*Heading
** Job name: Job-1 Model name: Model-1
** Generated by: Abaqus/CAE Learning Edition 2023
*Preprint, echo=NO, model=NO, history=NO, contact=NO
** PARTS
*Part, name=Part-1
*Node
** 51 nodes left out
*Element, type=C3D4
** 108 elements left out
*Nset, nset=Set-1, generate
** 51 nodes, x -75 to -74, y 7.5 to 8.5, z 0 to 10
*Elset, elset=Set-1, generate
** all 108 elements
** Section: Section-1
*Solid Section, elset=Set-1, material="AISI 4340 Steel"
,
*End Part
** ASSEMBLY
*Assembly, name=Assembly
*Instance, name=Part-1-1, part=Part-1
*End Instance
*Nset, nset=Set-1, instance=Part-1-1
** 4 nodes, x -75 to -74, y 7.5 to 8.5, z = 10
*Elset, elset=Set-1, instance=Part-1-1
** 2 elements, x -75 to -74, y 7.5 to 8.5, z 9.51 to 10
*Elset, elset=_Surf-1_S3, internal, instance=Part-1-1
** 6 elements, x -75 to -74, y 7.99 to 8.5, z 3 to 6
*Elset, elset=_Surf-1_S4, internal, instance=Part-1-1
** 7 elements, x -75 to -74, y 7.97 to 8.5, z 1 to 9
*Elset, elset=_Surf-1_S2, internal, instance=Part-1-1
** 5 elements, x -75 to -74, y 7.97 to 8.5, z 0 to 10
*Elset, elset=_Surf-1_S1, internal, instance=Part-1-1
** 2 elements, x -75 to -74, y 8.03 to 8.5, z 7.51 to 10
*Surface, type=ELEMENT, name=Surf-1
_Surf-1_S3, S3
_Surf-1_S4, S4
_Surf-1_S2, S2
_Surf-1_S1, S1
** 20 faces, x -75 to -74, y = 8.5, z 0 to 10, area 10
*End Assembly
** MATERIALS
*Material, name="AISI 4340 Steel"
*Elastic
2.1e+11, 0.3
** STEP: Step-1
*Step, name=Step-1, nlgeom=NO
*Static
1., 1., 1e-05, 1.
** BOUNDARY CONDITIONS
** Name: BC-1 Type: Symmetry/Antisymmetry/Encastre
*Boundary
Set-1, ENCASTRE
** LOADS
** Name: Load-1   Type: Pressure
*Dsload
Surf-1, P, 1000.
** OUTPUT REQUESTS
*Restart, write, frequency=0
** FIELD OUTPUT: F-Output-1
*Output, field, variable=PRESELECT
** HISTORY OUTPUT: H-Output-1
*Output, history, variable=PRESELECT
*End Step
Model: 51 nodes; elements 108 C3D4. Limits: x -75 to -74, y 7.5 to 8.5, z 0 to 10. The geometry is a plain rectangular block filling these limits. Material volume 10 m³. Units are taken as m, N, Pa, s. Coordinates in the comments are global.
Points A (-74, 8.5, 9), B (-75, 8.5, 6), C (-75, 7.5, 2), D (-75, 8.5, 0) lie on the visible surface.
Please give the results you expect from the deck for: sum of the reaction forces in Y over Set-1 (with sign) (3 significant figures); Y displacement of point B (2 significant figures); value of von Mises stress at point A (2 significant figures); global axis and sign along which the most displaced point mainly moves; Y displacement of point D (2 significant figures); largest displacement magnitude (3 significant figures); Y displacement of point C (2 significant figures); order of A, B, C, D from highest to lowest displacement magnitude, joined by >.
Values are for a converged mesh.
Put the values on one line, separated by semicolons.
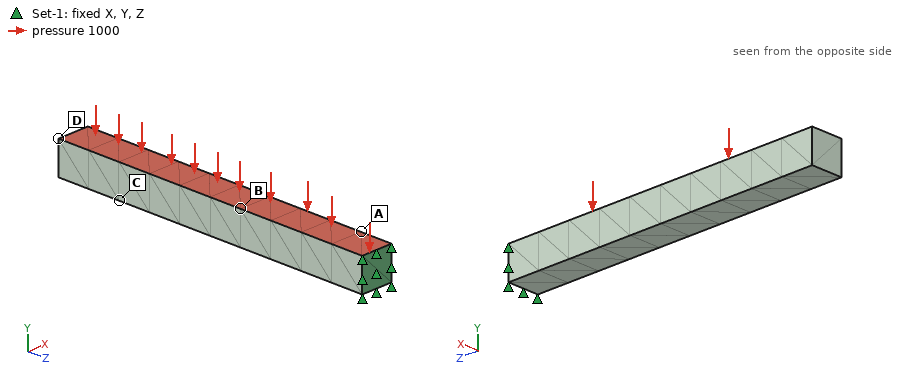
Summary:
10000 N; -1.7e-05 m; 2.4e+05 Pa; -Y; -7.1e-05 m; 7.15e-05 m; -5.2e-05 m; D > C > B > A
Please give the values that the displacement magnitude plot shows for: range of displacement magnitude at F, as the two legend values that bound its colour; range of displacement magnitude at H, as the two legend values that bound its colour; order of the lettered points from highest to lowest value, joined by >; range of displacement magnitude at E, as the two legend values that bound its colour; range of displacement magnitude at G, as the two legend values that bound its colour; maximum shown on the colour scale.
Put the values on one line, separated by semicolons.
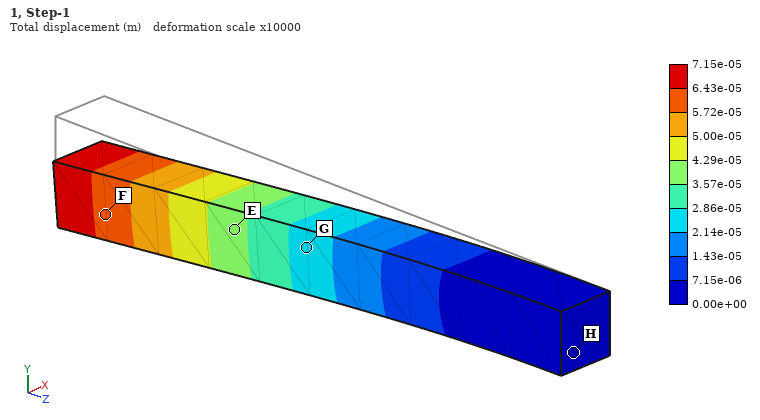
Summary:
5.72e-05 to 6.43e-05 m; 0.00e+00 to 7.15e-06 m; F > E > G > H; 3.57e-05 to 4.29e-05 m; 2.14e-05 to 2.86e-05 m; 7.15e-05 m
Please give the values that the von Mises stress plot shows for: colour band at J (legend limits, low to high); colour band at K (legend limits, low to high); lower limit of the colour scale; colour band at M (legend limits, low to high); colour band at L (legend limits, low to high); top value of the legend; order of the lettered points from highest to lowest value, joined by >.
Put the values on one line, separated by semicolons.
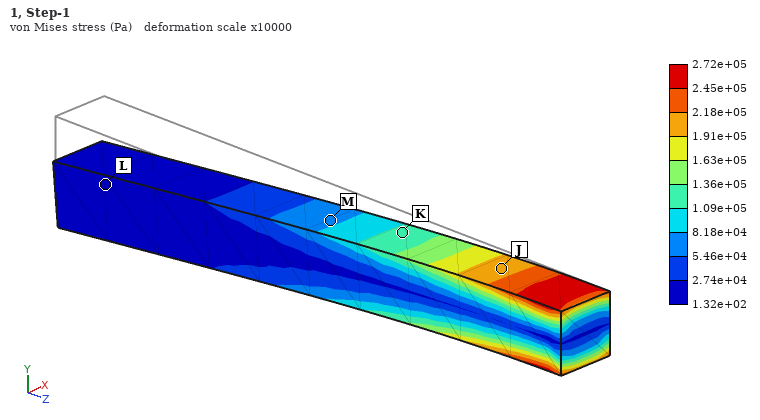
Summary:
1.91e+05 to 2.18e+05 Pa; 1.09e+05 to 1.36e+05 Pa; 1.32e+02 Pa; 5.46e+04 to 8.18e+04 Pa; 1.32e+02 to 2.74e+04 Pa; 2.72e+05 Pa; J > K > M > L
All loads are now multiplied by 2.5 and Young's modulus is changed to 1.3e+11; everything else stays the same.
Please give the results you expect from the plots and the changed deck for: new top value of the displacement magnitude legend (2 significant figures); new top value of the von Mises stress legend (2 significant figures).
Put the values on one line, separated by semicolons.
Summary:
2.9e-04 m; 6.8e+05 Pa
